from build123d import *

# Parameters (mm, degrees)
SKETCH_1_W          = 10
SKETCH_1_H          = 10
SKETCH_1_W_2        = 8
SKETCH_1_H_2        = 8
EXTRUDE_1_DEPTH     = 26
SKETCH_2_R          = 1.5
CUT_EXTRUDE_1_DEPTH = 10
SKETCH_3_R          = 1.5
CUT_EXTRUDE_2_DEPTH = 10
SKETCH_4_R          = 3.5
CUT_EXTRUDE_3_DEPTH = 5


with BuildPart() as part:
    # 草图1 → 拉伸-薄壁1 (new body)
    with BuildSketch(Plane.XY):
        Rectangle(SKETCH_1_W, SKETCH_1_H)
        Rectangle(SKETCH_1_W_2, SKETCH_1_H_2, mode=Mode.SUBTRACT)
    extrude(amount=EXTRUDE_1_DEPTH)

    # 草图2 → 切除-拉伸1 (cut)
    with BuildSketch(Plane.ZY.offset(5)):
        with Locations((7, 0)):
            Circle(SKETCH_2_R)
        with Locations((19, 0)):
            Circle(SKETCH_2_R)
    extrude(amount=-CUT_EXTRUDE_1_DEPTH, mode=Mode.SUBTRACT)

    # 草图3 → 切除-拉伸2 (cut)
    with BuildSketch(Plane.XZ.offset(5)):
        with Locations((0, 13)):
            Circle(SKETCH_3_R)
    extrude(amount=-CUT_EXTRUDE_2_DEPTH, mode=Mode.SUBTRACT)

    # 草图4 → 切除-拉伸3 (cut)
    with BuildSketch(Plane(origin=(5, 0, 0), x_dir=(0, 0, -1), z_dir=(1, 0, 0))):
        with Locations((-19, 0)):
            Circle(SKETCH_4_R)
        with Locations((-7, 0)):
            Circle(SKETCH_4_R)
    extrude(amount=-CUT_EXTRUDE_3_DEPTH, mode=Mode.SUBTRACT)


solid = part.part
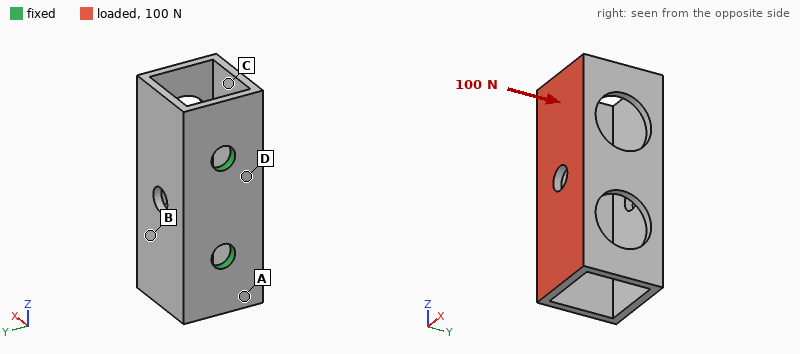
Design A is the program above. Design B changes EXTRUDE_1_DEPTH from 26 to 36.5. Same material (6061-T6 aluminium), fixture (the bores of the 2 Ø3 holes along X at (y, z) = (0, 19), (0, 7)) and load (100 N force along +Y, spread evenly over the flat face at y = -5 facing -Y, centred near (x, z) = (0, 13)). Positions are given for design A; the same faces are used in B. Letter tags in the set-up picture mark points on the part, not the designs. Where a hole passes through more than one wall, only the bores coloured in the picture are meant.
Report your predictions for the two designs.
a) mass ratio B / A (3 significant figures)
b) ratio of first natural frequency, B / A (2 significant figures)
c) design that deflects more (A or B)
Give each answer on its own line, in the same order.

1.46
0.87
A
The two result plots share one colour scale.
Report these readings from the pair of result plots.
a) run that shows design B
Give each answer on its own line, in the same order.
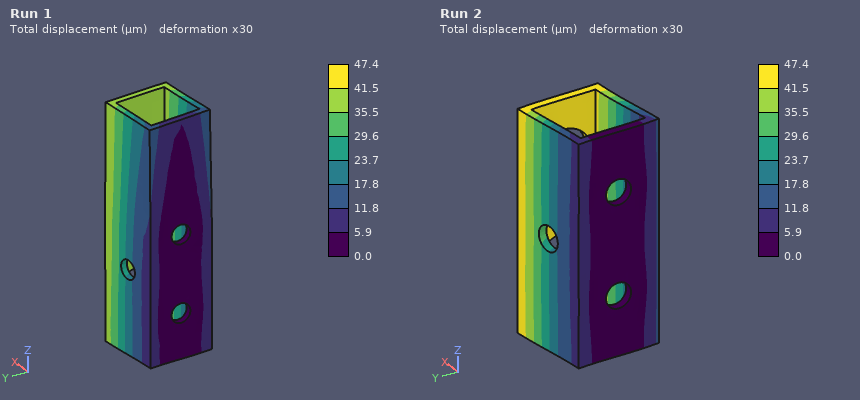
Run 1
